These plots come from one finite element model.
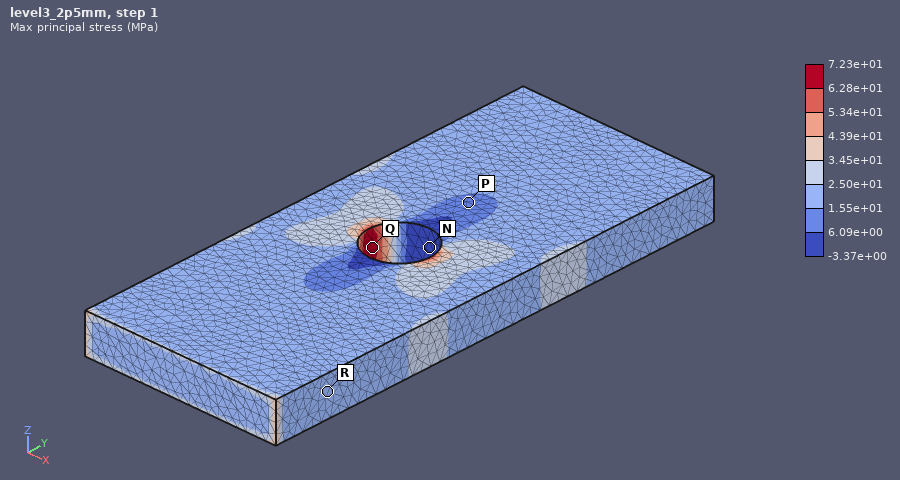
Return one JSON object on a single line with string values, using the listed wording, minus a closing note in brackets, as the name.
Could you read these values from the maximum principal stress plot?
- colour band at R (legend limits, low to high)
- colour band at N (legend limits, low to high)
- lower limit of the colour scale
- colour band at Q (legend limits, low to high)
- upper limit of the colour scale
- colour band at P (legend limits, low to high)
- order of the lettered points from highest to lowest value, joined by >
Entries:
{"colour band at R": "1.55e+01 to 2.50e+01 MPa", "colour band at N": "-3.37e+00 to 6.09e+00 MPa", "lower limit of the colour scale": "-3.37e+00 MPa", "colour band at Q": "6.28e+01 to 7.23e+01 MPa", "upper limit of the colour scale": "7.23e+01 MPa", "colour band at P": "6.09e+00 to 1.55e+01 MPa", "order of the lettered points from highest to lowest value, joined by >": "Q > R > P > N"}
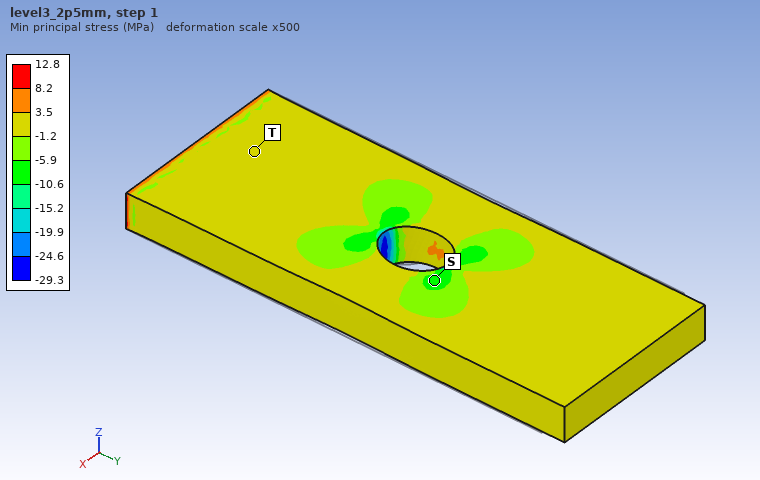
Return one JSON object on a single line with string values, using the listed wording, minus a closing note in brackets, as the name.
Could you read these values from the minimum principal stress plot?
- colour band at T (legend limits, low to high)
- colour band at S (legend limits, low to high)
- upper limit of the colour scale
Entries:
{"colour band at T": "-1.2 to 3.5 MPa", "colour band at S": "-10.6 to -5.9 MPa", "upper limit of the colour scale": "12.8 MPa"}
